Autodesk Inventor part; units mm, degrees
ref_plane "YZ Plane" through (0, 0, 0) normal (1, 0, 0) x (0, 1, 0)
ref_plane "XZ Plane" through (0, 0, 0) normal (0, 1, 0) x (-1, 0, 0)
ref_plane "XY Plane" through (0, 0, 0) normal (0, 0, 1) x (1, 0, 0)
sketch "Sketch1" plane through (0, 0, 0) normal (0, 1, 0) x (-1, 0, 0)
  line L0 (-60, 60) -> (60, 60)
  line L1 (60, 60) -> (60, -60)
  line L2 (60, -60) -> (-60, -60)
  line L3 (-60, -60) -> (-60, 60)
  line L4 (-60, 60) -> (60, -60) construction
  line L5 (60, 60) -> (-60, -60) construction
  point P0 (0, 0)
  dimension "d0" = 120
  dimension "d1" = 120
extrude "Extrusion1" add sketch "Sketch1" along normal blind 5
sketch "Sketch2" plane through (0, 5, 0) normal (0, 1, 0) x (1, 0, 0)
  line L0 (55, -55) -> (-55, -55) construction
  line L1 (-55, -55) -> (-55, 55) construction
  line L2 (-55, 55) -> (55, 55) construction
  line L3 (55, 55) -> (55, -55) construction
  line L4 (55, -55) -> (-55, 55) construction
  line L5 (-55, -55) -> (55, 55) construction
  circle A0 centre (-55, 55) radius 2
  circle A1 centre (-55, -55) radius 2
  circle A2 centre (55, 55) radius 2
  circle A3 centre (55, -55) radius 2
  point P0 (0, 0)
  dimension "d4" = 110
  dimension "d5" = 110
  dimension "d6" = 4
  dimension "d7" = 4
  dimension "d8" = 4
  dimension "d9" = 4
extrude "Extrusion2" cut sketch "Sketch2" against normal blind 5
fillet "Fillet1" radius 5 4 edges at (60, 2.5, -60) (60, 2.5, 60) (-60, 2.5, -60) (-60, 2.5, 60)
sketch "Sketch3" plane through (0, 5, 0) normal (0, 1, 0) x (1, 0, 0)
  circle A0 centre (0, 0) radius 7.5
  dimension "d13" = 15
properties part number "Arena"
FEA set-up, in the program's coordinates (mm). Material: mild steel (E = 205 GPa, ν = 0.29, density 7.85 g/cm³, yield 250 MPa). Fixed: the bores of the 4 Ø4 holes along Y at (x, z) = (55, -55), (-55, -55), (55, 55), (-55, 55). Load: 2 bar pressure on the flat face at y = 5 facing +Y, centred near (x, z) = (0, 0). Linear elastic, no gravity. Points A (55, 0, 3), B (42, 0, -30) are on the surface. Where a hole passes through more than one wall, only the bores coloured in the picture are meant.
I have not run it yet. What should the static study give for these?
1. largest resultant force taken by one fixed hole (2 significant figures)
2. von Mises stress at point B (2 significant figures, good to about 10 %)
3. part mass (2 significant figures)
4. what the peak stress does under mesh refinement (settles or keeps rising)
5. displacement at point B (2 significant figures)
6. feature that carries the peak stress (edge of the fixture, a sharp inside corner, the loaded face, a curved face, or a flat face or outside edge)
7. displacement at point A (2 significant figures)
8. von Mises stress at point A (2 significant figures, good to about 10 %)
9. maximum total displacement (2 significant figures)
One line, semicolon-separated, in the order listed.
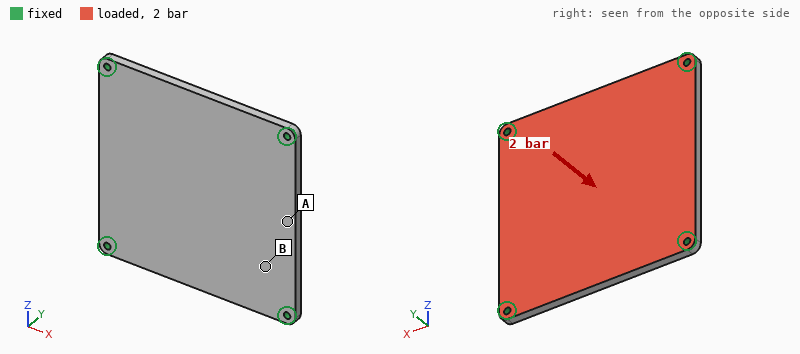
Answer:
720 N; 17 MPa; 560 g; keeps rising; 0.057 mm; edge of the fixture; 0.067 mm; 40 MPa; 0.12 mm
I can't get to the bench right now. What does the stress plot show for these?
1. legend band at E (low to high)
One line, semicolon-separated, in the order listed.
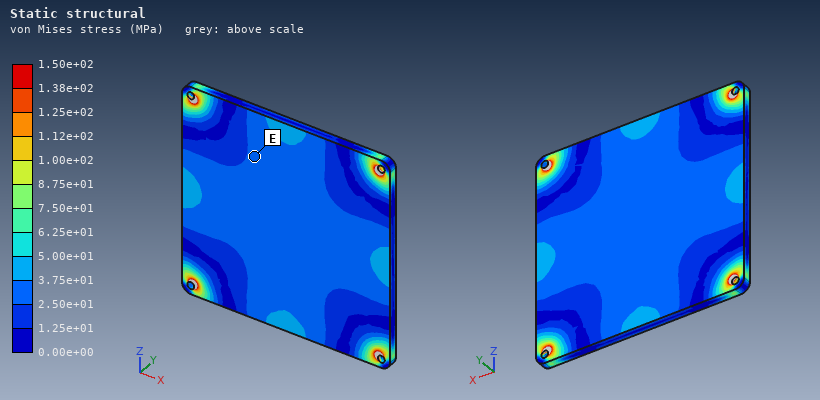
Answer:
2.50e+01 to 3.75e+01 MPa
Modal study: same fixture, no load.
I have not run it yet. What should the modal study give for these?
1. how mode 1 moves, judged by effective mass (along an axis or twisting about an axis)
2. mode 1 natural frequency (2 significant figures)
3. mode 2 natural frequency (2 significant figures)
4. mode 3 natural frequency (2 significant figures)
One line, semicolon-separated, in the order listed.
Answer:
along Y; 1200 Hz; 2300 Hz; 2300 Hz
